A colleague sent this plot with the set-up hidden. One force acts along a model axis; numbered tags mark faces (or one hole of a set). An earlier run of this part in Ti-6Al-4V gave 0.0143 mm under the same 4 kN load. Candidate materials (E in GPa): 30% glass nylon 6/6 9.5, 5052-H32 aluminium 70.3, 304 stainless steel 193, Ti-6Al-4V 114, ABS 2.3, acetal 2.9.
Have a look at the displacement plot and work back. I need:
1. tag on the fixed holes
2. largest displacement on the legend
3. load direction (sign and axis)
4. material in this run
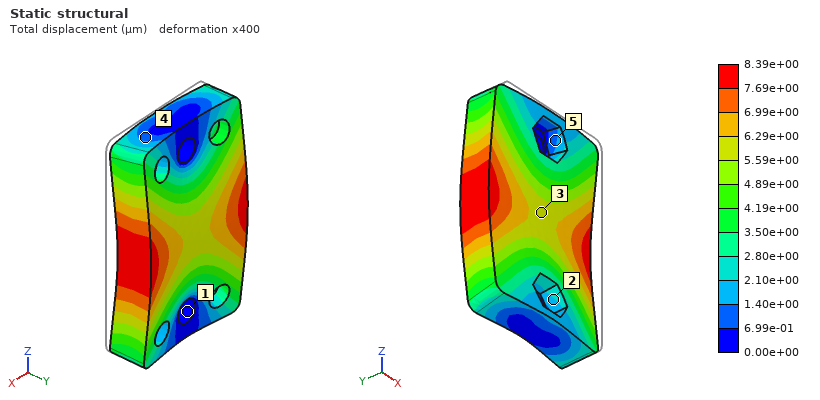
1
8.39e+00 µm
+Y
304 stainless steel
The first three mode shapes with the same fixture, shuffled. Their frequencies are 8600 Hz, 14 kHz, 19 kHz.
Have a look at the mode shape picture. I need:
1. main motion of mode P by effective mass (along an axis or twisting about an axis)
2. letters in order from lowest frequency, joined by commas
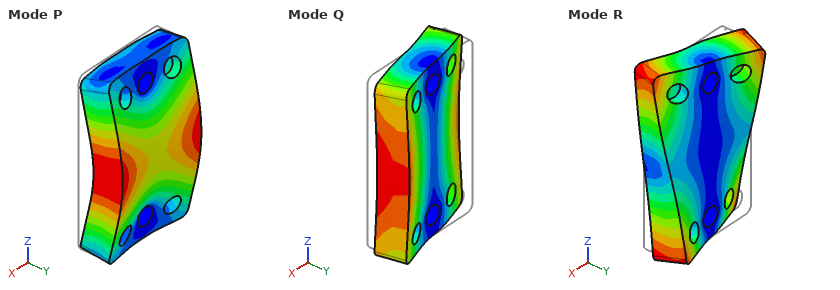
along Y
Q, P, R
